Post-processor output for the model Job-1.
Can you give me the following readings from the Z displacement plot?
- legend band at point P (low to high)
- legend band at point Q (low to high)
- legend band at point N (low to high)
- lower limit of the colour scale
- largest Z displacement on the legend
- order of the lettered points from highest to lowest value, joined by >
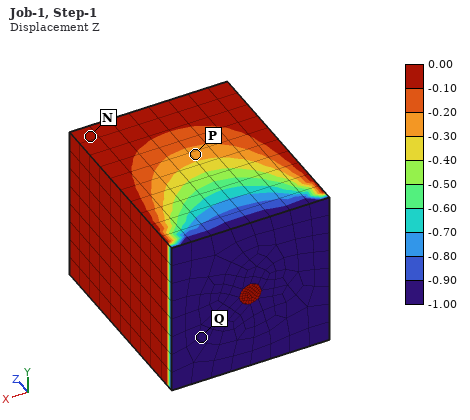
-0.30 to -0.20
-1.00 to -0.90
-0.10 to 0.00
-1.00
0.00
N > P > Q
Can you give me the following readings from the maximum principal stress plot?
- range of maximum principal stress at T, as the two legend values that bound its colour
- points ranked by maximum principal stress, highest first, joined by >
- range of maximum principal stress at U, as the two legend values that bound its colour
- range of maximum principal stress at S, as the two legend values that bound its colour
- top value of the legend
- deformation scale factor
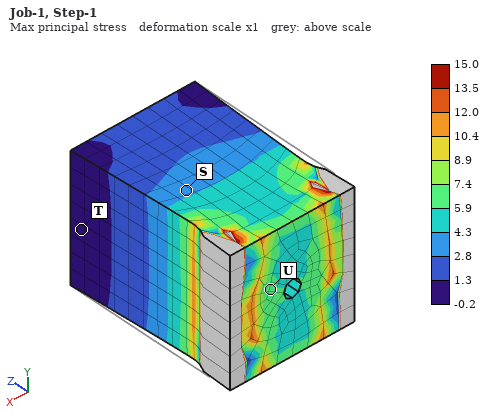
-0.2 to 1.3
U > S > T
5.9 to 7.4
2.8 to 4.3
15.0
1
